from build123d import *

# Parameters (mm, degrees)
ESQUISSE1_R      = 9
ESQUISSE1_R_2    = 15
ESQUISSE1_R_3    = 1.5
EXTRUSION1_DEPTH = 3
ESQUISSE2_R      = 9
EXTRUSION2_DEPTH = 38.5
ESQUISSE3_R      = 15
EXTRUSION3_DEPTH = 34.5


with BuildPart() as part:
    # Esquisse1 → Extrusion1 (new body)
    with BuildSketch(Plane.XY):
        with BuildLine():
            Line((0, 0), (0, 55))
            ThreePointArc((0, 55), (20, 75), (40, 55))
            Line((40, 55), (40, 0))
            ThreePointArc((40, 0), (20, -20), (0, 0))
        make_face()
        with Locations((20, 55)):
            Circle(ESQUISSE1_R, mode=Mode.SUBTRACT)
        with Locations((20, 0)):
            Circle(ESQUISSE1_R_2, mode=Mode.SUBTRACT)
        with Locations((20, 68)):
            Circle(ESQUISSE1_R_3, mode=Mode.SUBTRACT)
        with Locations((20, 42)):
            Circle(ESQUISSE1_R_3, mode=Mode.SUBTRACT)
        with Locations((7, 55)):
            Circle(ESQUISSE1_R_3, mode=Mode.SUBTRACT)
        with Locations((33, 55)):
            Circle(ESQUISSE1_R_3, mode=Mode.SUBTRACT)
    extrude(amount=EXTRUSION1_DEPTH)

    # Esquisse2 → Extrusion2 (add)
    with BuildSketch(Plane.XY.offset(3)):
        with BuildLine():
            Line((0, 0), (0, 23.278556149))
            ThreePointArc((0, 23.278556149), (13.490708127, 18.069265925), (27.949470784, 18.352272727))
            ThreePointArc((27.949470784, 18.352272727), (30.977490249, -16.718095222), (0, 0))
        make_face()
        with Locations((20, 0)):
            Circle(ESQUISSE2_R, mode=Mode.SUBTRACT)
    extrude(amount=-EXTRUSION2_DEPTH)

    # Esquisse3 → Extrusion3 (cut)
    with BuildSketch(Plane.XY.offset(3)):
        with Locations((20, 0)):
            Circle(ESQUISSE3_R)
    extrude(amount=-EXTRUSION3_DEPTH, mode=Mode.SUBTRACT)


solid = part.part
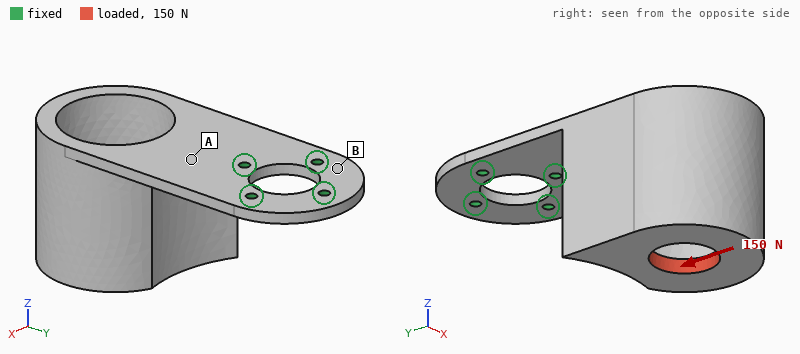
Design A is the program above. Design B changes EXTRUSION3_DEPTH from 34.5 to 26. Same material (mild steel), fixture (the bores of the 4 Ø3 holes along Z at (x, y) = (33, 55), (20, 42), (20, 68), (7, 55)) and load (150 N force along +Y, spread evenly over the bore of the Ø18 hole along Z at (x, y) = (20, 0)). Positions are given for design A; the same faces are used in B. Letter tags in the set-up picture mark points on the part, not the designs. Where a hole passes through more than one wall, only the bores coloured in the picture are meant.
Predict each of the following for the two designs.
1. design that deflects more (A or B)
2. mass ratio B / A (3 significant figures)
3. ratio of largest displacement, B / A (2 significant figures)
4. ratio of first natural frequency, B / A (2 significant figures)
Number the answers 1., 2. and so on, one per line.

1. A
2. 1.12
3. 0.88
4. 0.92
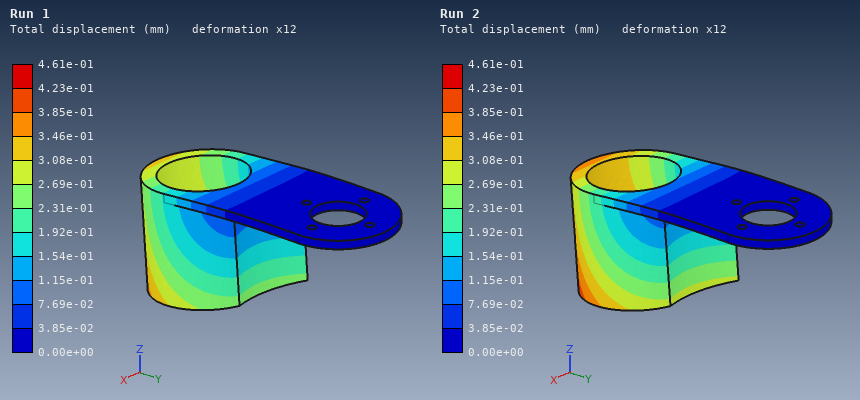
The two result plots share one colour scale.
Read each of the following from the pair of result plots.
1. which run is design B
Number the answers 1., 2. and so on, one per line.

1. Run 1
